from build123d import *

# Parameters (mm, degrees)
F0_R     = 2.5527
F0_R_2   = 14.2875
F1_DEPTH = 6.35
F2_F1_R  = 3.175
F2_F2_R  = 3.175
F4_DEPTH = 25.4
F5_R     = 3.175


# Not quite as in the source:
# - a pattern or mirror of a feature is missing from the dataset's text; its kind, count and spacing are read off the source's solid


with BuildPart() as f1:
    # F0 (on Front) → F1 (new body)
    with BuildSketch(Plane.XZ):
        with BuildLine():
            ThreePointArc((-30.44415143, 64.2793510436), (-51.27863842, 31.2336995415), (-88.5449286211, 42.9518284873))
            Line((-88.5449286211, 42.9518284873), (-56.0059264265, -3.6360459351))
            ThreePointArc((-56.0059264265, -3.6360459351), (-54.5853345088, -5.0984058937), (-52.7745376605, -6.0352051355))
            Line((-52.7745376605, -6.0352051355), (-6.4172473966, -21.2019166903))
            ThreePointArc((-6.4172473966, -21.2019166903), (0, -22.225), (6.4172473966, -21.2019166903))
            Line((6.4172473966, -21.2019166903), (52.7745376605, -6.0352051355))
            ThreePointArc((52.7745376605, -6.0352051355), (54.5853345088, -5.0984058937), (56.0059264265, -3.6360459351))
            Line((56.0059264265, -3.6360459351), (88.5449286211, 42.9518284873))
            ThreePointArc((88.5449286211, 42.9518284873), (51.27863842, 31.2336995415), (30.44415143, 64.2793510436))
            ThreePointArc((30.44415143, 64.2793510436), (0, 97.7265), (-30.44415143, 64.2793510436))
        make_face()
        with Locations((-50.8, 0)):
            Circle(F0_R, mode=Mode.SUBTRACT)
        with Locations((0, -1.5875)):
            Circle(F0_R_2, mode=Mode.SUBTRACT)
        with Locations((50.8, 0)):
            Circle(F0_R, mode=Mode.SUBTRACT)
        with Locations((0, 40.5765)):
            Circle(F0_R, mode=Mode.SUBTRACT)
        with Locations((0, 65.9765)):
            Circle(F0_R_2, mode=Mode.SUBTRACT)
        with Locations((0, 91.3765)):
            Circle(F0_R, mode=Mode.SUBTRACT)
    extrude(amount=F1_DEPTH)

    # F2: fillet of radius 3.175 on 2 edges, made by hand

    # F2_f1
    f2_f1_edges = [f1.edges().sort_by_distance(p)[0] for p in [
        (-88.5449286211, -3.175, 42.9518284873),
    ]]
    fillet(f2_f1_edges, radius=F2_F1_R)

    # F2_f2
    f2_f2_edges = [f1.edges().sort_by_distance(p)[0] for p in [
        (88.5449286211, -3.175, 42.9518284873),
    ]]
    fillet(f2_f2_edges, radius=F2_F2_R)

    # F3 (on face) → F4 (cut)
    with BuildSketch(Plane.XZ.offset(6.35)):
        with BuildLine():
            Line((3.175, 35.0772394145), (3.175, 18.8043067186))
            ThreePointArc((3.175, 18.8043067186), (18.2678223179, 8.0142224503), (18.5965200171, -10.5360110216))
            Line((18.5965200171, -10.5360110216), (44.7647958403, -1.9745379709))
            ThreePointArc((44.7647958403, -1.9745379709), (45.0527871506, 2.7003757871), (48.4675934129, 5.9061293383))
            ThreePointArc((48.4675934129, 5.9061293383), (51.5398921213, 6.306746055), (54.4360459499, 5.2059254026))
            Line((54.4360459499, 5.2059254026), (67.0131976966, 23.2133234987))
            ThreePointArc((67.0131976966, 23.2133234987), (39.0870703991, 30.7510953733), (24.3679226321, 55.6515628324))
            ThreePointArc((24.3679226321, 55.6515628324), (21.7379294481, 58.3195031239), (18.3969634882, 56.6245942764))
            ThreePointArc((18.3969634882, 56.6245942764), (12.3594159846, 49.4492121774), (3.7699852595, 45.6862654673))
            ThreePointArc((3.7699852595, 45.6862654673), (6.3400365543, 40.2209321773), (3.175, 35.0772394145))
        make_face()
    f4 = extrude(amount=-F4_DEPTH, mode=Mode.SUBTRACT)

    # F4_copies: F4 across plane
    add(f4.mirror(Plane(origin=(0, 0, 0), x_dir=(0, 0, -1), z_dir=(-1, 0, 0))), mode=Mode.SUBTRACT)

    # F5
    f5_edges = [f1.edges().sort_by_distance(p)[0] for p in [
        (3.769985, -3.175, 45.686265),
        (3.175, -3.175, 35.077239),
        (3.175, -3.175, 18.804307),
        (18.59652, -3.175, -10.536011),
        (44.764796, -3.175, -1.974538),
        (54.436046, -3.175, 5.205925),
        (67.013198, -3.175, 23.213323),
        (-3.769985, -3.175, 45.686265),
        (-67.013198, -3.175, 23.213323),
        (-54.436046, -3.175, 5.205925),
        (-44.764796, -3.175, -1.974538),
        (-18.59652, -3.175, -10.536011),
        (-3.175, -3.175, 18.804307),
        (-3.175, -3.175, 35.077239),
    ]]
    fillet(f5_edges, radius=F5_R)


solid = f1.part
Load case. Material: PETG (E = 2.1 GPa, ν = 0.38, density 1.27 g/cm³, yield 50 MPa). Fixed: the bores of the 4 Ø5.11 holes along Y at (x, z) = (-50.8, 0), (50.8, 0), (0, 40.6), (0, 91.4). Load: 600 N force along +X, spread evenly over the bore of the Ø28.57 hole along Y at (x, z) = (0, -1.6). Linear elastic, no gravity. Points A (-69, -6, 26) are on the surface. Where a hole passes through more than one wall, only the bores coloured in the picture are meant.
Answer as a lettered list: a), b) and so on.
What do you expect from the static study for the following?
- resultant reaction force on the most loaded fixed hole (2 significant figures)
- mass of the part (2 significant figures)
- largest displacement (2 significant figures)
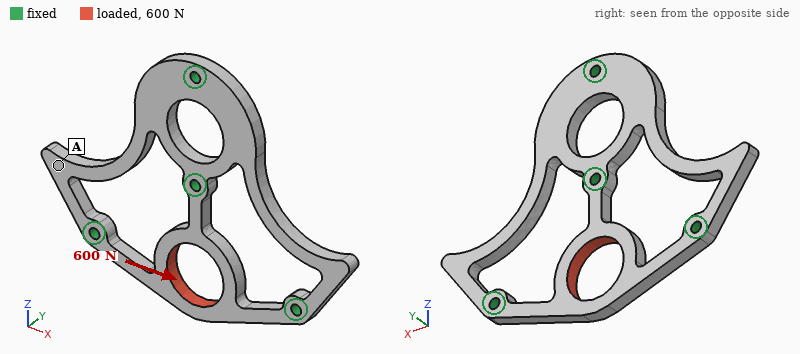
a) 220 N
b) 36 g
c) 0.64 mm
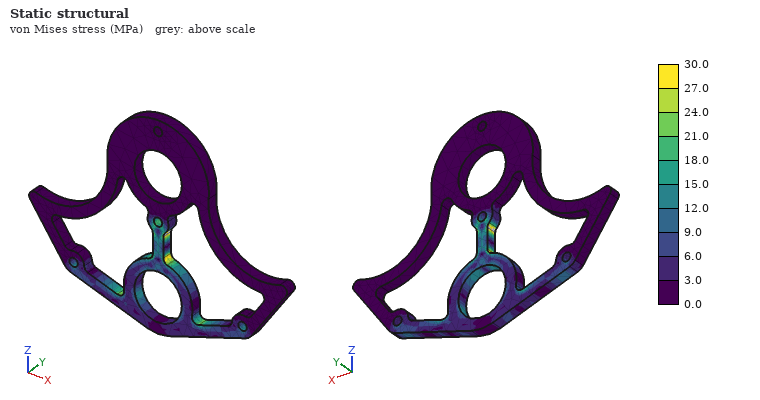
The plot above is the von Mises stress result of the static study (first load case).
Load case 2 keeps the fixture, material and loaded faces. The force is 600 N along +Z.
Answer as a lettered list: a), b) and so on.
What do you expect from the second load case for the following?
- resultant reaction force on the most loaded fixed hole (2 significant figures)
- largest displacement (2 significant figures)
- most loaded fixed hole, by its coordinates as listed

a) 420 N
b) 0.48 mm
c) (0, 40.6)
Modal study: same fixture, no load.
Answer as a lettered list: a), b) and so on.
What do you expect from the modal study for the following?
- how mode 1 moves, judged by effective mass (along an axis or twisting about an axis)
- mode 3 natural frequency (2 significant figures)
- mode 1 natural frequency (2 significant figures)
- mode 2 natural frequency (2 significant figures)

a) along Y
b) 740 Hz
c) 660 Hz
d) 710 Hz
